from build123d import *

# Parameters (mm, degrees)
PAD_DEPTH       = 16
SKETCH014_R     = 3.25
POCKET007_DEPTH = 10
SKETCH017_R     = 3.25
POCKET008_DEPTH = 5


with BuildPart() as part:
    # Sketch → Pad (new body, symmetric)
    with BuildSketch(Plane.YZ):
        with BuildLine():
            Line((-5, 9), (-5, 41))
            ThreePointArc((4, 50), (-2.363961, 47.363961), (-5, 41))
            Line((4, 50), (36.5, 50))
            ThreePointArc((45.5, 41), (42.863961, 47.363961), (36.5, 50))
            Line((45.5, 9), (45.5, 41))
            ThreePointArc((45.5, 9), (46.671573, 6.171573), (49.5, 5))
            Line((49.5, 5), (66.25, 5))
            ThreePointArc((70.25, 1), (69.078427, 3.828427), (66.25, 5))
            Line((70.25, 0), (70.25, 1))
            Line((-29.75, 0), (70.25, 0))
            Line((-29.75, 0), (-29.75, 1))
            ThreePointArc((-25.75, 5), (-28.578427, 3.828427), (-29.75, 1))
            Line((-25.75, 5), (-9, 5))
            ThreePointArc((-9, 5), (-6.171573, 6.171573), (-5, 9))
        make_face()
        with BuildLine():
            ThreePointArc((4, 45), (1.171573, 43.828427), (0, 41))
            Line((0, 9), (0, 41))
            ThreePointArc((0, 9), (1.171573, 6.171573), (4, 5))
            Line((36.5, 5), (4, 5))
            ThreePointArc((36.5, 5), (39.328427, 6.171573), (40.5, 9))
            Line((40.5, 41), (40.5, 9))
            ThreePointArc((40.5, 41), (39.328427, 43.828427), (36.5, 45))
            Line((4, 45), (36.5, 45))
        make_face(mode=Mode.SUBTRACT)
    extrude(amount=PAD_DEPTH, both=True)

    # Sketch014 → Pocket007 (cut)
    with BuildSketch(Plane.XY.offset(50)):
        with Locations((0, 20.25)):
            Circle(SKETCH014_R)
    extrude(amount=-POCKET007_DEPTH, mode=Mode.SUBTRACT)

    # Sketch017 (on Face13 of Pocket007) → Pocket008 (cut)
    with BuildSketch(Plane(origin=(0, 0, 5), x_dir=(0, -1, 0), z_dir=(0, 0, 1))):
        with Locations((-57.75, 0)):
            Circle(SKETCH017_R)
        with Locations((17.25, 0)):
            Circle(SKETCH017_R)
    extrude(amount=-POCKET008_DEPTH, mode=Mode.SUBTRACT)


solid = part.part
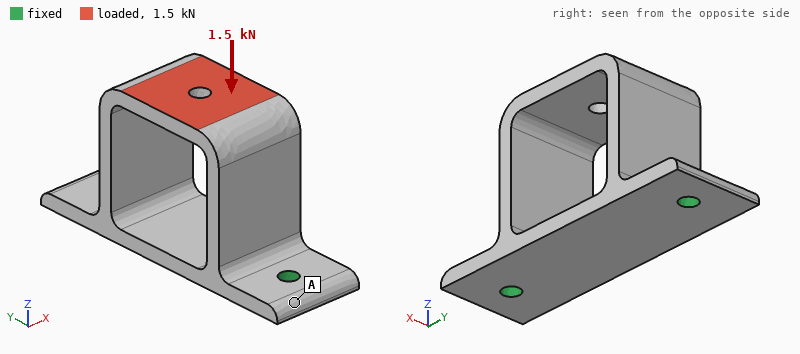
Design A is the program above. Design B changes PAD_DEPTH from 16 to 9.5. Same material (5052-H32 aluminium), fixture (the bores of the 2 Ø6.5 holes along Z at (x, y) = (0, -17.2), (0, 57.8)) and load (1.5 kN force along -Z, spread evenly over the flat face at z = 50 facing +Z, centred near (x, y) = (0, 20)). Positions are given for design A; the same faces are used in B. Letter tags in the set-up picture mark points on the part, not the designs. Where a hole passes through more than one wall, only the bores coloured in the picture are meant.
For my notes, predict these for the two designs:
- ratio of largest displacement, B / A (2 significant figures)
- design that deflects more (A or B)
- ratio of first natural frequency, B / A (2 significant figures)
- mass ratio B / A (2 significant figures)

1.6
B
1.0
0.59
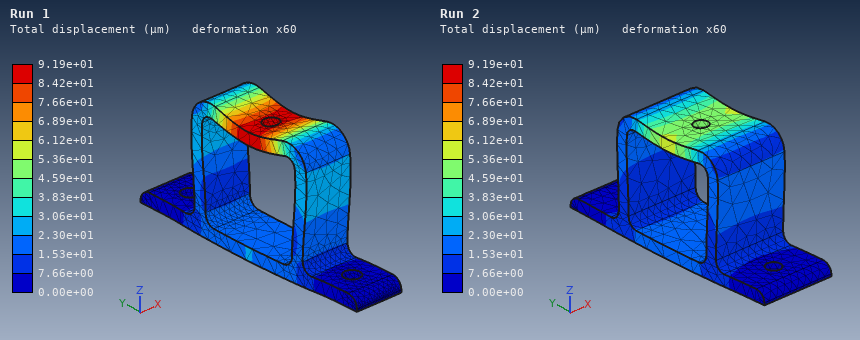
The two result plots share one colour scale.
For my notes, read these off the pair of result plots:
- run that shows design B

Run 1
